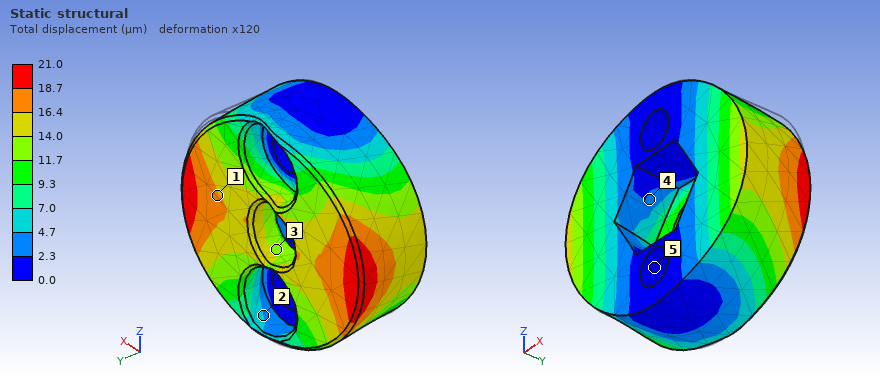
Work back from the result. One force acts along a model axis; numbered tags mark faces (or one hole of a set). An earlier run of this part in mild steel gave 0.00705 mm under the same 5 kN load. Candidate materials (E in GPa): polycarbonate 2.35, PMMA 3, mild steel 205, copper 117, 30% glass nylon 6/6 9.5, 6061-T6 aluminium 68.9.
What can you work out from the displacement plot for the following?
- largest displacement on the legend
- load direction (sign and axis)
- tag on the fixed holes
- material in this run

21.0 µm
-X
5
6061-T6 aluminium
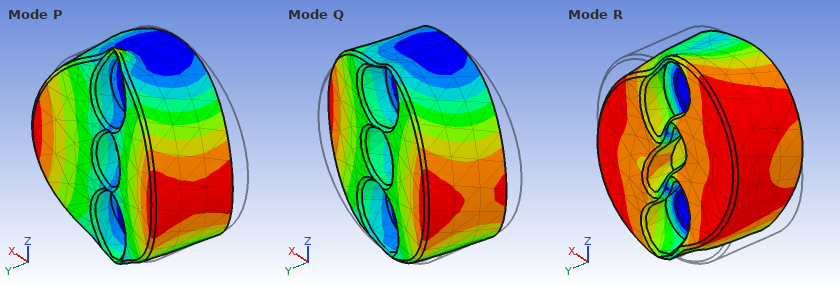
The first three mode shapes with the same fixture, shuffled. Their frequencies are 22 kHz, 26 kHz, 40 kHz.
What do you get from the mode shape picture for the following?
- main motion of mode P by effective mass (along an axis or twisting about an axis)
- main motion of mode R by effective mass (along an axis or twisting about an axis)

along Y
twisting about Y
